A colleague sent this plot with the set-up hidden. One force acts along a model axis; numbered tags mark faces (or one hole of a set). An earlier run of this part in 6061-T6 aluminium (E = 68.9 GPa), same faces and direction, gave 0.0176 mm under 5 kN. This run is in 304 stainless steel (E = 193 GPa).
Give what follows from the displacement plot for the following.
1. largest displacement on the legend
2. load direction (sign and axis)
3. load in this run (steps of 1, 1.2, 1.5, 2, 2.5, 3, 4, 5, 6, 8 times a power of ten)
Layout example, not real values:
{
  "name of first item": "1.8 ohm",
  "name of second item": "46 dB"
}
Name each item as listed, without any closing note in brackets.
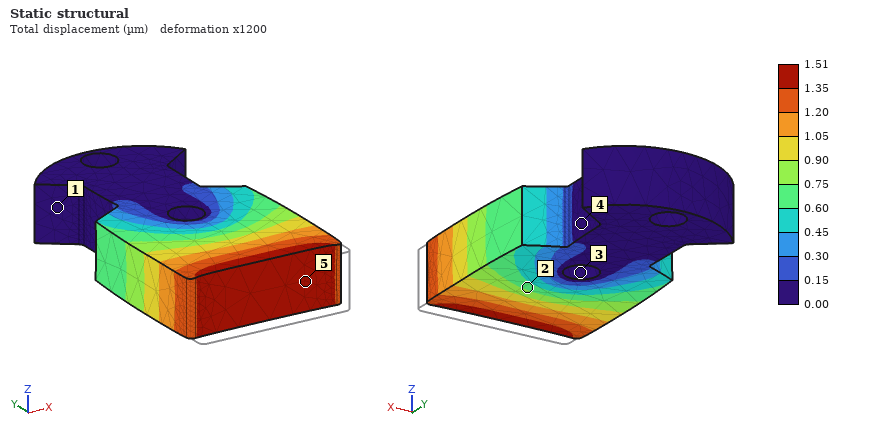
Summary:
{
  "largest displacement on the legend": "1.51 µm",
  "load direction": "+Y",
  "load in this run": "1.2 kN"
}
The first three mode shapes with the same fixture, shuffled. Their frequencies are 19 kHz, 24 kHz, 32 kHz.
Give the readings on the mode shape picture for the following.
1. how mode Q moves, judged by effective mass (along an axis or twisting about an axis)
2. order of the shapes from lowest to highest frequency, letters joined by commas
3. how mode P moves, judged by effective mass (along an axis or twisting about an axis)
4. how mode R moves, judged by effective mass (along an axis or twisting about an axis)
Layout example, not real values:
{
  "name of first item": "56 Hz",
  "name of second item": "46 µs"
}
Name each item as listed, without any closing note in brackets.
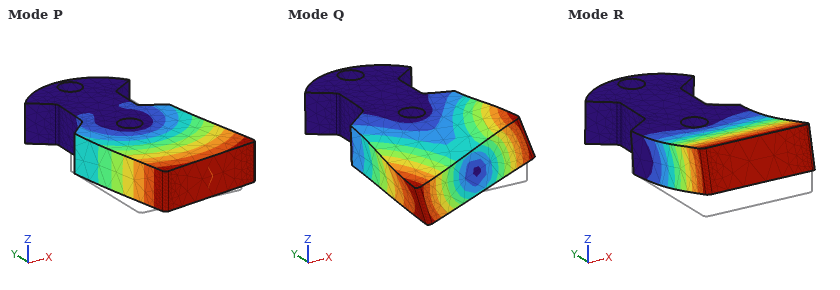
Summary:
{
  "how mode Q moves, judged by effective mass": "twisting about Y",
  "order of the shapes from lowest to highest frequency, letters joined by commas": "R, P, Q",
  "how mode P moves, judged by effective mass": "along X",
  "how mode R moves, judged by effective mass": "along Z"
}
